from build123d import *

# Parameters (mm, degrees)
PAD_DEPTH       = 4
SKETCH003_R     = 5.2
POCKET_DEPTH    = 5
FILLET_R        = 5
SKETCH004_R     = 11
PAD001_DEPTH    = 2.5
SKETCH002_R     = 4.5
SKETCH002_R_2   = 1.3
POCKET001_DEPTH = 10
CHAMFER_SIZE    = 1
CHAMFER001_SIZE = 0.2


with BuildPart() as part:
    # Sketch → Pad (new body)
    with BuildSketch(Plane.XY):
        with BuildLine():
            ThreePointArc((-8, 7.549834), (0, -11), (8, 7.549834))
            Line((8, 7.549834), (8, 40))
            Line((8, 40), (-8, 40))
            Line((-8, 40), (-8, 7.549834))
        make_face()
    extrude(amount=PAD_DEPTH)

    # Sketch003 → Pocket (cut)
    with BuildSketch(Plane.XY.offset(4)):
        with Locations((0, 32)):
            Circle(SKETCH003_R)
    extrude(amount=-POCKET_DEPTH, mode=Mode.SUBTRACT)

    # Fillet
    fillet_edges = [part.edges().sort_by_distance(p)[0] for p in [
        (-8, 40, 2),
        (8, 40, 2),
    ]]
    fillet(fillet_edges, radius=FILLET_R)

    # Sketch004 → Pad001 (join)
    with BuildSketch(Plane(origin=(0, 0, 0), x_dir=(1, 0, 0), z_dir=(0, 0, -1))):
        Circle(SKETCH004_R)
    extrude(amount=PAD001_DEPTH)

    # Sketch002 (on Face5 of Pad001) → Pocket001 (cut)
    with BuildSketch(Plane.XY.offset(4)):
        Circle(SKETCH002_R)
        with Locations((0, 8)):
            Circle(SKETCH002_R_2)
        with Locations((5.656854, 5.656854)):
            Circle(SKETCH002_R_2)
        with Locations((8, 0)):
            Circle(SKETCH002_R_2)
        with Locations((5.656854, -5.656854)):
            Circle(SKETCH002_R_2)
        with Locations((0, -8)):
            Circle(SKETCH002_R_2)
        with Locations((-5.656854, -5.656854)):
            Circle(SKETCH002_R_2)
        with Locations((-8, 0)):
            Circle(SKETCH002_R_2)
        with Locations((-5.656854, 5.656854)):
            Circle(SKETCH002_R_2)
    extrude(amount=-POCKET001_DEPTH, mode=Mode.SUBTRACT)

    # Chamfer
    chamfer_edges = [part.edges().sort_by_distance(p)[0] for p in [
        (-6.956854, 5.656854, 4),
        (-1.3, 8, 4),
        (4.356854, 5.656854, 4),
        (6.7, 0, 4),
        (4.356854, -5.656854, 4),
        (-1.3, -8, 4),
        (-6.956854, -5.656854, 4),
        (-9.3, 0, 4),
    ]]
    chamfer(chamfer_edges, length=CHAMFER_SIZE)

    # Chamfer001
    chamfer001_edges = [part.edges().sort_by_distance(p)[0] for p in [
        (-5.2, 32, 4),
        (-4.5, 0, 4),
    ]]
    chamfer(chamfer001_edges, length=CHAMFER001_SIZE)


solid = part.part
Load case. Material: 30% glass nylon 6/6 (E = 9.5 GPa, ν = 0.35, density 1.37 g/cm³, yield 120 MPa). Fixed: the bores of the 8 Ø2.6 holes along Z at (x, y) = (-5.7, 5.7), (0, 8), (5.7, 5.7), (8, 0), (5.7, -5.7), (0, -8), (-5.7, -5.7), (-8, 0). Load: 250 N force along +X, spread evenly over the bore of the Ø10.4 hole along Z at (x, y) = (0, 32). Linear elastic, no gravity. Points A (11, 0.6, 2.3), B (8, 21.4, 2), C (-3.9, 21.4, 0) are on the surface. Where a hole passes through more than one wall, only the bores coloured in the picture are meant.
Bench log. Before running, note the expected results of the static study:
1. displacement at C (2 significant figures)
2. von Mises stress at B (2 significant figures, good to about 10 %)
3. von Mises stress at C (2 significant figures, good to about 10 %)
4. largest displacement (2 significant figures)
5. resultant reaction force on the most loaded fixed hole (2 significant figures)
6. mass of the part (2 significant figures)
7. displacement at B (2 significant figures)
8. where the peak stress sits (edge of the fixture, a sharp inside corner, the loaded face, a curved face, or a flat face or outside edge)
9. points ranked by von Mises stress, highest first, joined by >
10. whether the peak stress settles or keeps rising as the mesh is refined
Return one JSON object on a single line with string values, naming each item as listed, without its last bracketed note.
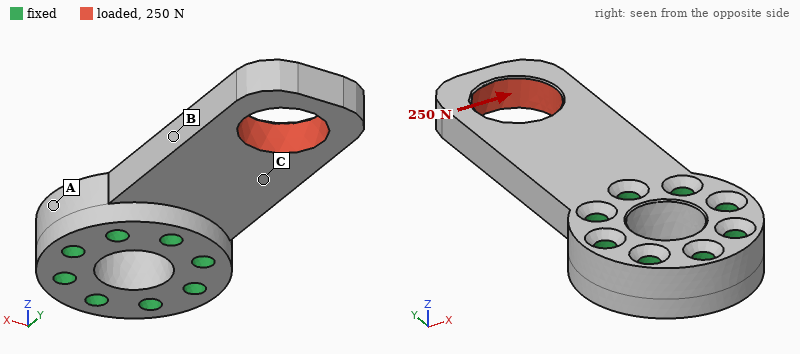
{"displacement at C": "0.064 mm", "von Mises stress at B": "18 MPa", "von Mises stress at C": "9.0 MPa", "largest displacement": "0.26 mm", "resultant reaction force on the most loaded fixed hole": "430 N", "mass of the part": "4.5 g", "displacement at B": "0.075 mm", "where the peak stress sits": "edge of the fixture", "points ranked by von Mises stress, highest first, joined by >": "B > C > A", "whether the peak stress settles or keeps rising as the mesh is refined": "keeps rising"}
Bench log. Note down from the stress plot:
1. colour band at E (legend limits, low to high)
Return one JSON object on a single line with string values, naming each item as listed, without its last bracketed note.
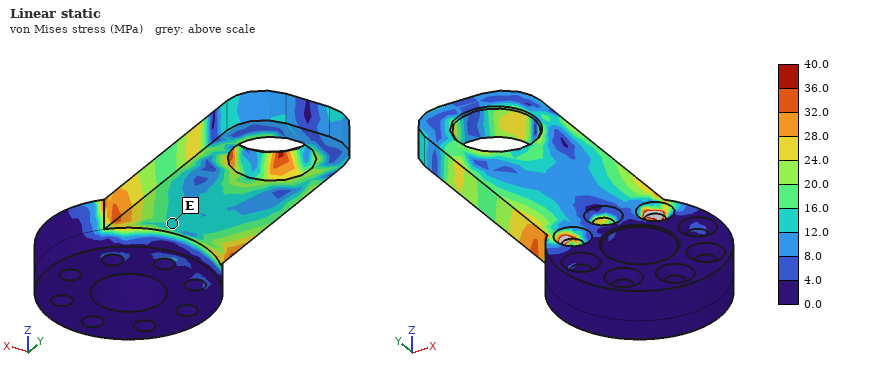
{"colour band at E": "12.0 to 16.0 MPa"}
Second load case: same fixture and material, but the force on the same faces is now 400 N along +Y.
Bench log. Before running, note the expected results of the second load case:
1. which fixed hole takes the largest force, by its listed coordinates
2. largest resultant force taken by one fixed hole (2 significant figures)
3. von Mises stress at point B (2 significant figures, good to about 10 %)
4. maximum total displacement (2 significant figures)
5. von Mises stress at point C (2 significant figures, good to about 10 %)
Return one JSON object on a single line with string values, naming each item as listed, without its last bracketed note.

{"which fixed hole takes the largest force, by its listed coordinates": "(0, 8)", "largest resultant force taken by one fixed hole": "160 N", "von Mises stress at point B": "10 MPa", "maximum total displacement": "46 µm", "von Mises stress at point C": "7.0 MPa"}
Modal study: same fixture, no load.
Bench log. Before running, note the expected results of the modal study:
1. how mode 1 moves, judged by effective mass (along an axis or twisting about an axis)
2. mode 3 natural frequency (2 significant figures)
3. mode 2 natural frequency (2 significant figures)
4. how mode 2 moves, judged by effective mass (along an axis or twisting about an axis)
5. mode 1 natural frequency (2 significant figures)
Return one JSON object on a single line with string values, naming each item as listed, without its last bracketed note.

{"how mode 1 moves, judged by effective mass": "along Z", "mode 3 natural frequency": "6300 Hz", "mode 2 natural frequency": "5900 Hz", "how mode 2 moves, judged by effective mass": "along X", "mode 1 natural frequency": "2100 Hz"}
